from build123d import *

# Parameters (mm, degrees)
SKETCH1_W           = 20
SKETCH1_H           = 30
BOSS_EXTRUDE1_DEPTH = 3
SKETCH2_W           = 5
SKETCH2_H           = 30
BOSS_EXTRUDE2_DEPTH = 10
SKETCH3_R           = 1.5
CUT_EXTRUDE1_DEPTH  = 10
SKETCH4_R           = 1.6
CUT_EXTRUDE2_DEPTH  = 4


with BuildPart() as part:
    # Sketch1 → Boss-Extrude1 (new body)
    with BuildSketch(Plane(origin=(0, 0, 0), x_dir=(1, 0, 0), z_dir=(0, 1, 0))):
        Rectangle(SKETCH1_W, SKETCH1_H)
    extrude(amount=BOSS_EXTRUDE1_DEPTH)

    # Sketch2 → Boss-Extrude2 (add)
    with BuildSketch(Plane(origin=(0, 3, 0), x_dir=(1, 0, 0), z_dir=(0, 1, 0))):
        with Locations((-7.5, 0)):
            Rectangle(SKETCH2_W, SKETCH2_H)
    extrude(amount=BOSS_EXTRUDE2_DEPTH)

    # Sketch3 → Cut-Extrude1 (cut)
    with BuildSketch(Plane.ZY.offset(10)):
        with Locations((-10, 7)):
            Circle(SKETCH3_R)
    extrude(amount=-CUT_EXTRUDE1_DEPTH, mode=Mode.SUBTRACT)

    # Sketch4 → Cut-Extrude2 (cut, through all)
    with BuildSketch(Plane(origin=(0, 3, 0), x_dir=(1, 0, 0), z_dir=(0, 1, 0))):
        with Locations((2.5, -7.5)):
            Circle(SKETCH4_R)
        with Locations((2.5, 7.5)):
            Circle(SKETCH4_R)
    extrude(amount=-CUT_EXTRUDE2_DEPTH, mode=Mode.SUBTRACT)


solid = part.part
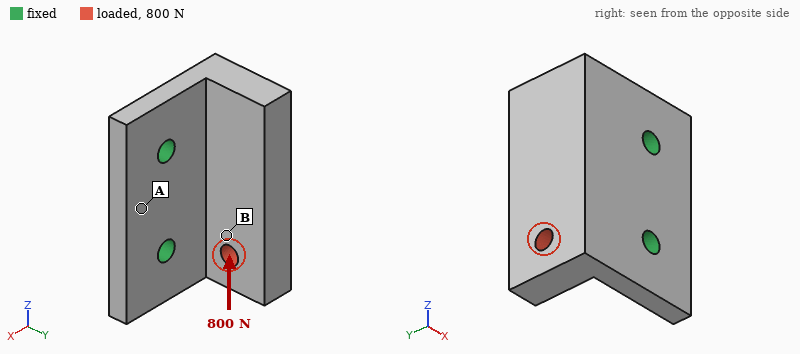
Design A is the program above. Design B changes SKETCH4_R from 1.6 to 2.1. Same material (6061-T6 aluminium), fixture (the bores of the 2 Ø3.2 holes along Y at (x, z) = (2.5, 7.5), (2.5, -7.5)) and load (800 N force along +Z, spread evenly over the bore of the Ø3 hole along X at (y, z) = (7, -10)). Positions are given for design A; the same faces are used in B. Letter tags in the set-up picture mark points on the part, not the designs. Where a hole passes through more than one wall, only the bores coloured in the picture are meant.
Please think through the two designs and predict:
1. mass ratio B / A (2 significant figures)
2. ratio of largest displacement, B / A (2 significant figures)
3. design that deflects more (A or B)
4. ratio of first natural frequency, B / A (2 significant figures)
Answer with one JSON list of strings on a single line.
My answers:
["0.99", "0.86", "A", "1.1"]
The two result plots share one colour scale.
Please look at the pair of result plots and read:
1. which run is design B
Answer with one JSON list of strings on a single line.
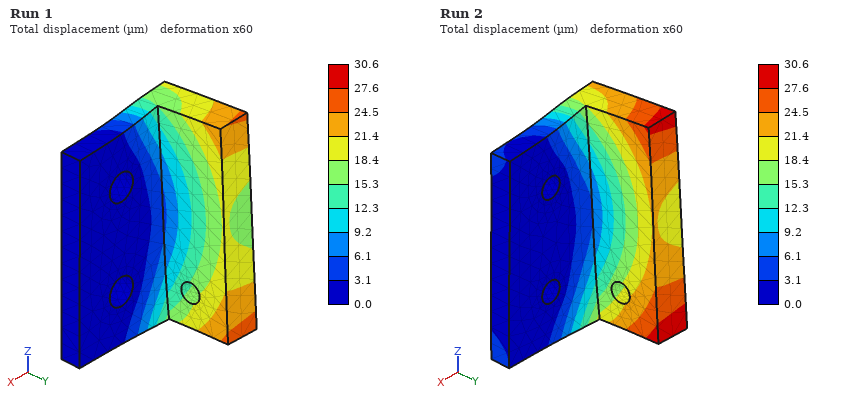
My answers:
["Run 1"]
